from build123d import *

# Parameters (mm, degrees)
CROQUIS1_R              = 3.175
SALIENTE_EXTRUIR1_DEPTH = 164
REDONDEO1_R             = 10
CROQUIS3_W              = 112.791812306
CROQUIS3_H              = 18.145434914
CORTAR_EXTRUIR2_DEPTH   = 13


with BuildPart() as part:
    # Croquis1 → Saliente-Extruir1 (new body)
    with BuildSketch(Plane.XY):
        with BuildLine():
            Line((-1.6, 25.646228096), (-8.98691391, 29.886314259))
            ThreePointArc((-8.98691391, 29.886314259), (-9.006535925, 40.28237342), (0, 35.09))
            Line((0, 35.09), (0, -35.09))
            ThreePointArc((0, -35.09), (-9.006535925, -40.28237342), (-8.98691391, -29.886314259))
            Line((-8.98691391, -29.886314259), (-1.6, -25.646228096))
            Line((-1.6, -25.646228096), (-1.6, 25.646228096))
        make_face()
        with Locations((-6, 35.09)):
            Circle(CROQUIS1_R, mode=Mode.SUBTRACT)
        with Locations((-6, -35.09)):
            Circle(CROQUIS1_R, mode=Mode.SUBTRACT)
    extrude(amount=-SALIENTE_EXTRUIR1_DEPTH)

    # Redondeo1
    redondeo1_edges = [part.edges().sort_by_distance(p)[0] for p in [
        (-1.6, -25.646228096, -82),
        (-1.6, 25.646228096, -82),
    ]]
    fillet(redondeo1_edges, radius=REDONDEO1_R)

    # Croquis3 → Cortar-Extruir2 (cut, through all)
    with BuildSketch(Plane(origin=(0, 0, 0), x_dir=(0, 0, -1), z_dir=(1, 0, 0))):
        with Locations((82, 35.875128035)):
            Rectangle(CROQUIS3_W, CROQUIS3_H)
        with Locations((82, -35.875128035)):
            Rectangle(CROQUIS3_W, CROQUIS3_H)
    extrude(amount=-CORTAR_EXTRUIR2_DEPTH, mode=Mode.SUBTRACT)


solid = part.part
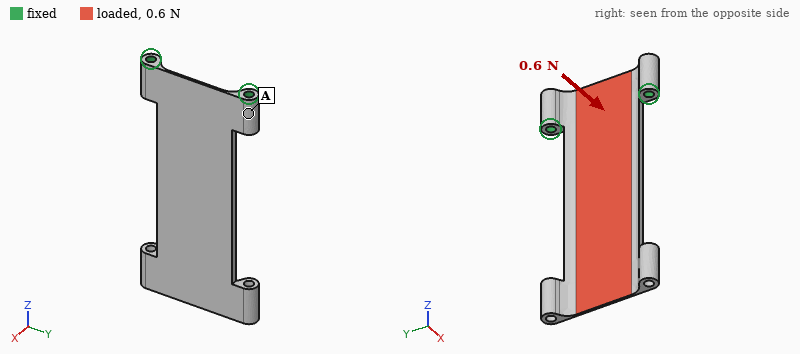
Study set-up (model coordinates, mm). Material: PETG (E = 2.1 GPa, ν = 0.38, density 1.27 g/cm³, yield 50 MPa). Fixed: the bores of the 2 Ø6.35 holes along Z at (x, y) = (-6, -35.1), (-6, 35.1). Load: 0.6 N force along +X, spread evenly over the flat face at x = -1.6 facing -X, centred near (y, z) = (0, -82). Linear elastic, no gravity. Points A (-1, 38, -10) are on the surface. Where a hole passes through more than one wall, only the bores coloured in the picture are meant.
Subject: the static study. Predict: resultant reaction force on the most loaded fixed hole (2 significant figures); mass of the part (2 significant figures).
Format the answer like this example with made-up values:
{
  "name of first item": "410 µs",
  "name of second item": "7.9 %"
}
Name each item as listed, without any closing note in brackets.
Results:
{
  "resultant reaction force on the most loaded fixed hole": "0.46 N",
  "mass of the part": "34 g"
}
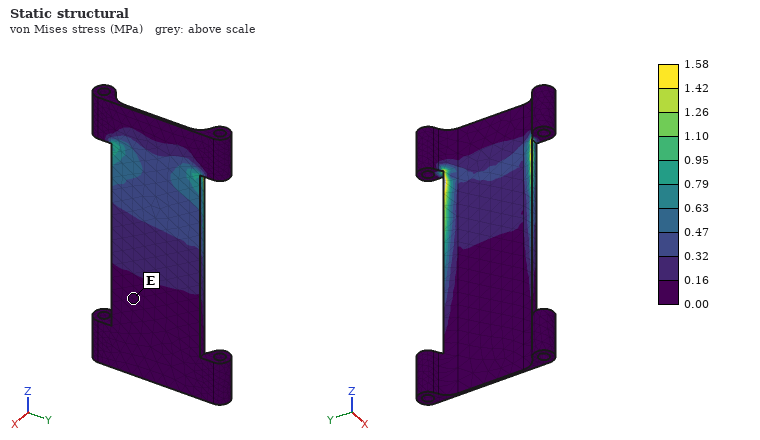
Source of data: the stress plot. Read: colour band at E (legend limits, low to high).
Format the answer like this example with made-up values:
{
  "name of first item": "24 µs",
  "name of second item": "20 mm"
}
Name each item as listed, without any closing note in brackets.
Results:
{
  "colour band at E": "0.00 to 0.16 MPa"
}
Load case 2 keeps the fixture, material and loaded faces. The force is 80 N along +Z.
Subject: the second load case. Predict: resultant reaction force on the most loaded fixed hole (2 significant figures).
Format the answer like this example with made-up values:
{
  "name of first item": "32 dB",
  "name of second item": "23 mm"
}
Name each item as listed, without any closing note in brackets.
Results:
{
  "resultant reaction force on the most loaded fixed hole": "41 N"
}
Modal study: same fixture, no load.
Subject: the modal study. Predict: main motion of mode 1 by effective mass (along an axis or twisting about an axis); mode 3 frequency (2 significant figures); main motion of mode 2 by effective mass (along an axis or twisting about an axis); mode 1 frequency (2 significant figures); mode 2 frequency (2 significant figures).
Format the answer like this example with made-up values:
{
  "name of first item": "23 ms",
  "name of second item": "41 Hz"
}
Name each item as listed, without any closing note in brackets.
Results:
{
  "main motion of mode 1 by effective mass": "along X",
  "mode 3 frequency": "140 Hz",
  "main motion of mode 2 by effective mass": "twisting about Z",
  "mode 1 frequency": "18 Hz",
  "mode 2 frequency": "48 Hz"
}
